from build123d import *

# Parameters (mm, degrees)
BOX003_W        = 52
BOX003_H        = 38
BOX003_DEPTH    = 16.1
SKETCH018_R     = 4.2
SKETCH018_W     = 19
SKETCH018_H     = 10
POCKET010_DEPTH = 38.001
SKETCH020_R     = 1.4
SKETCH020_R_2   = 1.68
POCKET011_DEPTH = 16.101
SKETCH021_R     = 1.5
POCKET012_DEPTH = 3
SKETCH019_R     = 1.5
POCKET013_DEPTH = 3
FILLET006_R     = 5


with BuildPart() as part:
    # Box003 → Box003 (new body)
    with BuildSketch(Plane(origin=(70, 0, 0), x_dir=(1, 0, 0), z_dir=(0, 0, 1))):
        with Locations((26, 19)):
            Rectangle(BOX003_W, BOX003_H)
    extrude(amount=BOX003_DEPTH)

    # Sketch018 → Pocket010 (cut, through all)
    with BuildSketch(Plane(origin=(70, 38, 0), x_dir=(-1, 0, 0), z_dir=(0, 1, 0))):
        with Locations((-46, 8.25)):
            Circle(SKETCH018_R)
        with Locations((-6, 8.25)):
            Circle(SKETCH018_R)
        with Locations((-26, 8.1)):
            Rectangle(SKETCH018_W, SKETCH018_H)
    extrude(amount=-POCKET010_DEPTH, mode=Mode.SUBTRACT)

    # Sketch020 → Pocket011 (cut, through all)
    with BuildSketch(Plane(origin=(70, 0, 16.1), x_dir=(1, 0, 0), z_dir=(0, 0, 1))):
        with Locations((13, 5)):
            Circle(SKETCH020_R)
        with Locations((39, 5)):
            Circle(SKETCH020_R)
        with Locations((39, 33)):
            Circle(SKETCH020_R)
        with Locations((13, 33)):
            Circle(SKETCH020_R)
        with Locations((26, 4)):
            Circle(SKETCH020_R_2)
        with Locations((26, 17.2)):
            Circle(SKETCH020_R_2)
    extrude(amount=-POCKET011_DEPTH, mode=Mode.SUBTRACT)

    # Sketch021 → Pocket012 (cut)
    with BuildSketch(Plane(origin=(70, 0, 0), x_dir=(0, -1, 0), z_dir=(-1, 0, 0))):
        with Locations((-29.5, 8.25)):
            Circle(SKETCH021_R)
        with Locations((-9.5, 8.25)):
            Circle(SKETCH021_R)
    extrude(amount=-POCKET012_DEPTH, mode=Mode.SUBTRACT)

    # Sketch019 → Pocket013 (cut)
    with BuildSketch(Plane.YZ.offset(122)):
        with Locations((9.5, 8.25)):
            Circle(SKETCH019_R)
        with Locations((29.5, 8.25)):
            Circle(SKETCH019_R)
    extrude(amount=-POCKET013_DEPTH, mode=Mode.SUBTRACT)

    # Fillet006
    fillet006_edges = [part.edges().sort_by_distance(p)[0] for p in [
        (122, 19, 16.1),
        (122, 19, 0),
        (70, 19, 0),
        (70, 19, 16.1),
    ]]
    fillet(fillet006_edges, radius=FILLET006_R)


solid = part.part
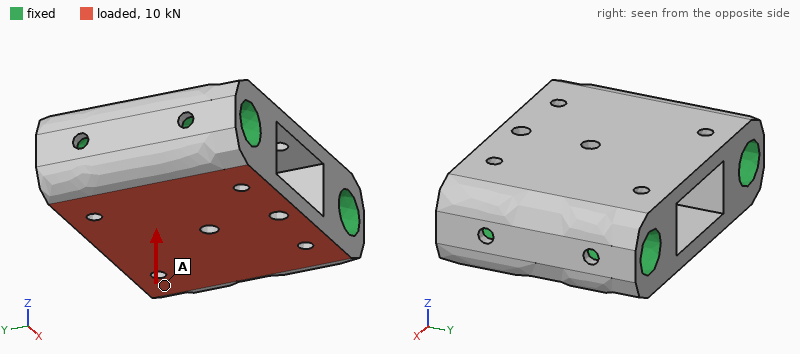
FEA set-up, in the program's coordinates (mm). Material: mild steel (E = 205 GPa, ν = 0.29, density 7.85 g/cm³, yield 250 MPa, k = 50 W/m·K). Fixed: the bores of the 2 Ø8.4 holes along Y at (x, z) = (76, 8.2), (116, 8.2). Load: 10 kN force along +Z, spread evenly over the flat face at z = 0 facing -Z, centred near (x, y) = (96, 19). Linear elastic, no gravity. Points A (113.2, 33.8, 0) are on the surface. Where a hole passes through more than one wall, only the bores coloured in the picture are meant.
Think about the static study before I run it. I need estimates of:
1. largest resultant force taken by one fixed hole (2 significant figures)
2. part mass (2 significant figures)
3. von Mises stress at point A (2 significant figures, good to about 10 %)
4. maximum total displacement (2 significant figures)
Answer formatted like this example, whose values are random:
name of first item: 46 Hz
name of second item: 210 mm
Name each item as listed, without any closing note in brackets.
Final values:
largest resultant force taken by one fixed hole: 5.1 kN
part mass: 150 g
von Mises stress at point A: 15 MPa
maximum total displacement: 12 µm
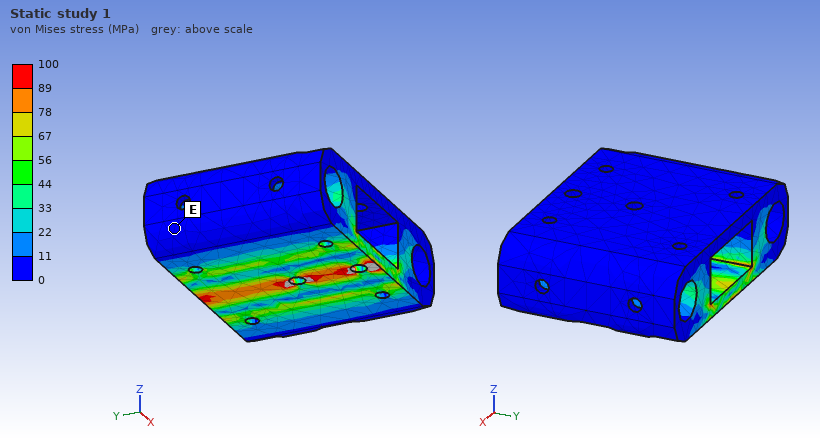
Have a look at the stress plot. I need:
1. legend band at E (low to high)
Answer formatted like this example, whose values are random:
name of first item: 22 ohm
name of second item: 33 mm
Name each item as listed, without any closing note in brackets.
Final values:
legend band at E: 0 to 11 MPa
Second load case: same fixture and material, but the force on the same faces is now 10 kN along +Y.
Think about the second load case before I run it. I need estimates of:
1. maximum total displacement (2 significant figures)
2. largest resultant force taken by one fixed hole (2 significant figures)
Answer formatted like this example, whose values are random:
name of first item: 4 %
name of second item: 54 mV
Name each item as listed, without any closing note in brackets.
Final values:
maximum total displacement: 5.8 µm
largest resultant force taken by one fixed hole: 5.0 kN
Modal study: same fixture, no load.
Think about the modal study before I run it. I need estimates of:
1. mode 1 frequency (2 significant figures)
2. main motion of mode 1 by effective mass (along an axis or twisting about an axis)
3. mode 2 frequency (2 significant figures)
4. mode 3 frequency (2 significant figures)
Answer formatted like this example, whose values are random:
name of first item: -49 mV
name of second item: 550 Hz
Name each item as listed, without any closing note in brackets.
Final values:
mode 1 frequency: 28 kHz
main motion of mode 1 by effective mass: along Z
mode 2 frequency: 29 kHz
mode 3 frequency: 29 kHz
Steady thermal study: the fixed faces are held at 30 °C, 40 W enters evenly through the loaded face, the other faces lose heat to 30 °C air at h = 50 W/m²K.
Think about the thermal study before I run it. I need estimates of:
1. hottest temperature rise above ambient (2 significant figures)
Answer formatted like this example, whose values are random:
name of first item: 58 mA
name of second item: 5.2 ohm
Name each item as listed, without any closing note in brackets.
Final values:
hottest temperature rise above ambient: 17 K
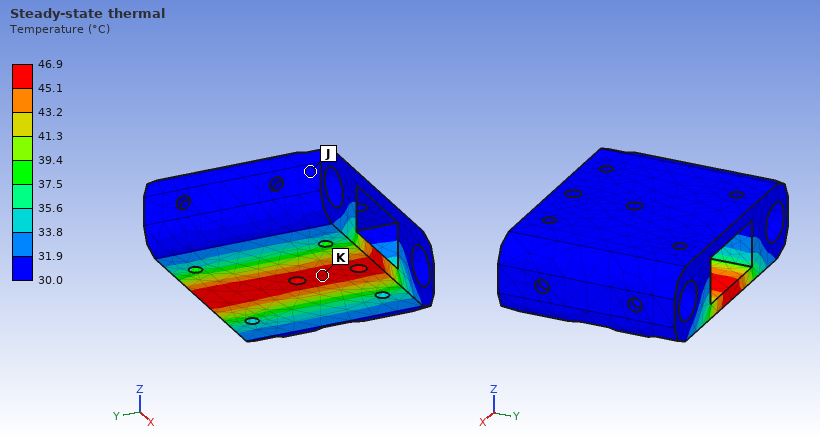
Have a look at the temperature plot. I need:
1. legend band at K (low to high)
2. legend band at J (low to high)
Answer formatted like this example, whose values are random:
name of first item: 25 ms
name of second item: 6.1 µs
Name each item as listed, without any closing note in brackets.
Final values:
legend band at K: 45.1 to 46.9 °C
legend band at J: 30.0 to 31.9 °C
